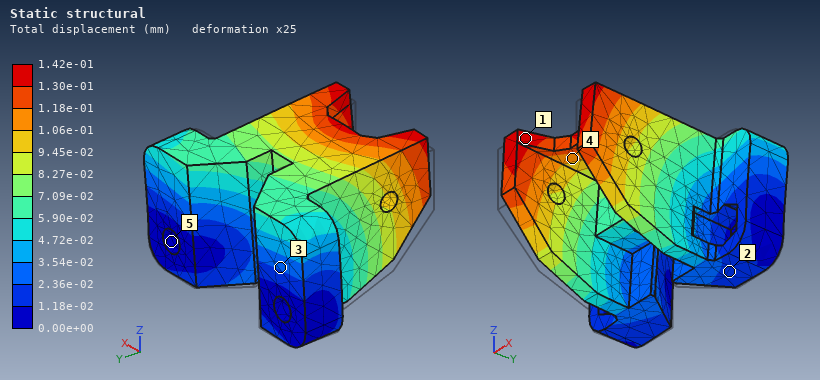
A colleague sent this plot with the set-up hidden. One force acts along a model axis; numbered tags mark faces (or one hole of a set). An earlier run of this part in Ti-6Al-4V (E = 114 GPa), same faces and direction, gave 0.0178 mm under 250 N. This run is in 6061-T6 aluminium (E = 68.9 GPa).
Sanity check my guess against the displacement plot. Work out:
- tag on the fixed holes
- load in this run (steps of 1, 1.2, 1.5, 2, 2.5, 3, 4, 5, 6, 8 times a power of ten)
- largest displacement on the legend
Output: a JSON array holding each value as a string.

["5", "1.2 kN", "1.42e-01 mm"]
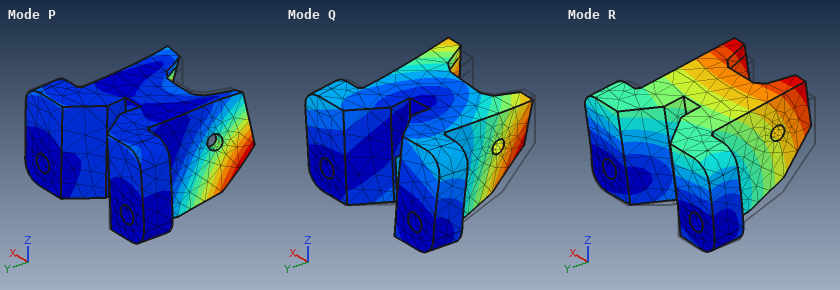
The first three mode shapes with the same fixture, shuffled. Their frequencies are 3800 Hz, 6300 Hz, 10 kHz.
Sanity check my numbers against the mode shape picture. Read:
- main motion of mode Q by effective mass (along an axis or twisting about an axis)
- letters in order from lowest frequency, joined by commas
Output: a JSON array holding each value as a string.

["along X", "R, Q, P"]
